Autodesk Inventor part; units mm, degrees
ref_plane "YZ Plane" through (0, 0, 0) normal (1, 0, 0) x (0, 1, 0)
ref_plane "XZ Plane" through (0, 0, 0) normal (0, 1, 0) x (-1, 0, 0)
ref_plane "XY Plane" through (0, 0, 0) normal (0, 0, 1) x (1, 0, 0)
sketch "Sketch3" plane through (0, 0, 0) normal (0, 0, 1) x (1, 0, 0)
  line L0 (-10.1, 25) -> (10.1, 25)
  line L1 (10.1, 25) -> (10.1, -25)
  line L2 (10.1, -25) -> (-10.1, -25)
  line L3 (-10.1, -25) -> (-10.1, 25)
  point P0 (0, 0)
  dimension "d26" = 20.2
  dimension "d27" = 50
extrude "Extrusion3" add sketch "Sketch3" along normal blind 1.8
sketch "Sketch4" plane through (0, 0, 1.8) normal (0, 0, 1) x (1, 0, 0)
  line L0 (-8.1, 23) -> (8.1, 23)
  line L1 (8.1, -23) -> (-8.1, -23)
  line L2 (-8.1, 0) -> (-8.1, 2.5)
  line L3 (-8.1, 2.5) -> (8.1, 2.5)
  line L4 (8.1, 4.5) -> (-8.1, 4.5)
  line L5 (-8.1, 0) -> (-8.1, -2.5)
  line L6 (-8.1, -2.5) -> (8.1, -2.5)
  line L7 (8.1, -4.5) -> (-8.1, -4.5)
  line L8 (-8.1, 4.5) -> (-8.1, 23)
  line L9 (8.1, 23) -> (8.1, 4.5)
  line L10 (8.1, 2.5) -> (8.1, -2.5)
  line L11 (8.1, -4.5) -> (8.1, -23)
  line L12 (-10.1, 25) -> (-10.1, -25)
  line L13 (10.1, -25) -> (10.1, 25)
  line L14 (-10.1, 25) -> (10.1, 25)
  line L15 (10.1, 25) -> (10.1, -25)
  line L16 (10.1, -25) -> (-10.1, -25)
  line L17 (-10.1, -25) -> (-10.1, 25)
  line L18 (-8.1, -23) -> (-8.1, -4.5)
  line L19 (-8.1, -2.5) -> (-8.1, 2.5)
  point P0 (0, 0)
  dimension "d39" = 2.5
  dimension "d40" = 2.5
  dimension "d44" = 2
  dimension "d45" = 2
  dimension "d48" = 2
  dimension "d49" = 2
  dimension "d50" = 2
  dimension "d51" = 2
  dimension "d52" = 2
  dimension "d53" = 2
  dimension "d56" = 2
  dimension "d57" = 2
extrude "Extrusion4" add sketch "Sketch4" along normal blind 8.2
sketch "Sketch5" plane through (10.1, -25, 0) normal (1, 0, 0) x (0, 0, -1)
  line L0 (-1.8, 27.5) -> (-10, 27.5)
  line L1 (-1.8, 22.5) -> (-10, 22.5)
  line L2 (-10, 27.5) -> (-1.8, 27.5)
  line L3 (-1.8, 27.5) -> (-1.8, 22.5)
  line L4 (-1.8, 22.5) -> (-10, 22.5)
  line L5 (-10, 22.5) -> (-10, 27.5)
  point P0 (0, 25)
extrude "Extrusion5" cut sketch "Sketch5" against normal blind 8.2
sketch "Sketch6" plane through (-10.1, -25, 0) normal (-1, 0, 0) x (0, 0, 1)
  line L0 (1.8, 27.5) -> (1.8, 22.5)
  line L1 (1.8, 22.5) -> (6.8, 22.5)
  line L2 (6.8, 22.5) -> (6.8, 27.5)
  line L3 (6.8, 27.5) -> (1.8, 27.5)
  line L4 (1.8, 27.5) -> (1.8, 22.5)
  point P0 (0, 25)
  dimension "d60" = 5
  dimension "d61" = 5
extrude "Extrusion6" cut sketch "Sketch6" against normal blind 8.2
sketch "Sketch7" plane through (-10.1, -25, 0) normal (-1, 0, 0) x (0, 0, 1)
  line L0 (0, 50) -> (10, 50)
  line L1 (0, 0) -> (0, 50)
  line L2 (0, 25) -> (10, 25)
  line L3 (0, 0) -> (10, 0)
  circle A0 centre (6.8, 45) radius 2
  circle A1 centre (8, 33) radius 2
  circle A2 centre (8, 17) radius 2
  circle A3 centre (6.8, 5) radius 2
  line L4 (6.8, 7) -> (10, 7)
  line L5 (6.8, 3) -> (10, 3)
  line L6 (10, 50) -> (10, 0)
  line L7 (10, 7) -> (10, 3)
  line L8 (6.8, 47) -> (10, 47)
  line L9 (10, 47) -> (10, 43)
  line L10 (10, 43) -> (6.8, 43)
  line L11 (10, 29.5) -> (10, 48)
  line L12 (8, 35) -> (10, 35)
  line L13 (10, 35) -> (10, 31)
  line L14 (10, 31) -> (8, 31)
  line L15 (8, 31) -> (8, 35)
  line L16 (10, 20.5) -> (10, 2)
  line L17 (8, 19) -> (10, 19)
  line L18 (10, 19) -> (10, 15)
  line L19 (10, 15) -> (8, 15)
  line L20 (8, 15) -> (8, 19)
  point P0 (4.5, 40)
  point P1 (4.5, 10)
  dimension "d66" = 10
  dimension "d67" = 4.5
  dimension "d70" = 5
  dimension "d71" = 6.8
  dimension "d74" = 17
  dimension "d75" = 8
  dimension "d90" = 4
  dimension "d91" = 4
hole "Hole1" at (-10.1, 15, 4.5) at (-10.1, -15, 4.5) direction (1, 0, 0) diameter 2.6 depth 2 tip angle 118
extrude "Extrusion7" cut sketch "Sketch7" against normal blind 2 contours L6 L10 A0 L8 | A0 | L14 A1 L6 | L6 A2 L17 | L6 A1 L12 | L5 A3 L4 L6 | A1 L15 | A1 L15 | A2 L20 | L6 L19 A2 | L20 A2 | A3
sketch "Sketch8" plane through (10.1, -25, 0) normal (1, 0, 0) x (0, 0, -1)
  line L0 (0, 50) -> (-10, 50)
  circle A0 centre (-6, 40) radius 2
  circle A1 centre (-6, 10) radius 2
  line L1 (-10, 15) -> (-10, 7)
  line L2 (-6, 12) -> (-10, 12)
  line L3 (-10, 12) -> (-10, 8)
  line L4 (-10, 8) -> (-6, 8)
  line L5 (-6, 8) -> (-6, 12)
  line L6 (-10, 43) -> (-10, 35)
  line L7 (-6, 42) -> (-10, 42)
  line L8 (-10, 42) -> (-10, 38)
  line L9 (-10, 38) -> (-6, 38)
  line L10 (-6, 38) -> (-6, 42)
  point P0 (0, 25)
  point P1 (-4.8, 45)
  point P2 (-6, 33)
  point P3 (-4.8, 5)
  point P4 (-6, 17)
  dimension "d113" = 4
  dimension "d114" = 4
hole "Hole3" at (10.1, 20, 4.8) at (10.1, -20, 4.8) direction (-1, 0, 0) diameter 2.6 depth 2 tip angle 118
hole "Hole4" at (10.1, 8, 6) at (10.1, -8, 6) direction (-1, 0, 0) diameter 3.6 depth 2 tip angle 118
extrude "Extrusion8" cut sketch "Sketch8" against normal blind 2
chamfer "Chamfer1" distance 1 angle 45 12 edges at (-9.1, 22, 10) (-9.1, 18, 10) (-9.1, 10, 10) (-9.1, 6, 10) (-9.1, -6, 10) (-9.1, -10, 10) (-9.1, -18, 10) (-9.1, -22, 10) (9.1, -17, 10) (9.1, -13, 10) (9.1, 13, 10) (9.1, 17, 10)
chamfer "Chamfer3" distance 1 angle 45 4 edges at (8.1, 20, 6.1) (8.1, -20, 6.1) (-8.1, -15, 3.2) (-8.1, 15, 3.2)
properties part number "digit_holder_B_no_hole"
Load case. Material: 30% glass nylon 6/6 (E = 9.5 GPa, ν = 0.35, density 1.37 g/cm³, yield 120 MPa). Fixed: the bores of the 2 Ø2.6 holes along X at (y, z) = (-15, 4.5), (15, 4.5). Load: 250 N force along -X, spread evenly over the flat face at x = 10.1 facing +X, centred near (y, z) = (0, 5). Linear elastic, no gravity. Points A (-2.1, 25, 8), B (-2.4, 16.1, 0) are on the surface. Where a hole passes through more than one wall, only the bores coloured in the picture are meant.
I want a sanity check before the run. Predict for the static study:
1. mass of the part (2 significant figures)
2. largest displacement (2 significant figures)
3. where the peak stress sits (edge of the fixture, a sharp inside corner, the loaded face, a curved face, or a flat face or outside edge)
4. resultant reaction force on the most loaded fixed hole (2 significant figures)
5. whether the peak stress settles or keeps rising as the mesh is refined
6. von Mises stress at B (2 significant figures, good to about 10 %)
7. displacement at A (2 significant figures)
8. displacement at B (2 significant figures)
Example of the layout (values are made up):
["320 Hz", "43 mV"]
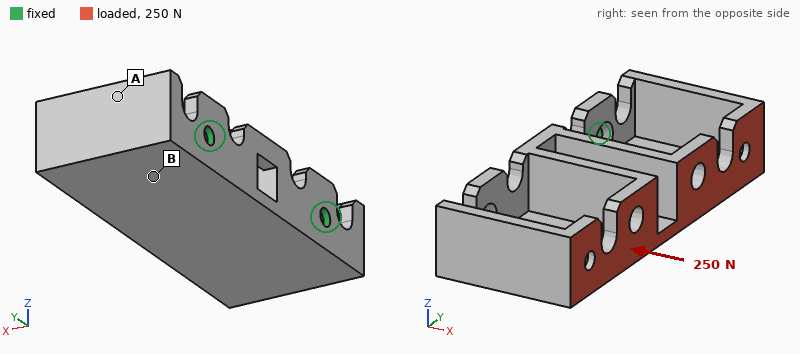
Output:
["5.5 g", "0.39 mm", "edge of the fixture", "130 N", "keeps rising", "7.1 MPa", "0.16 mm", "0.089 mm"]
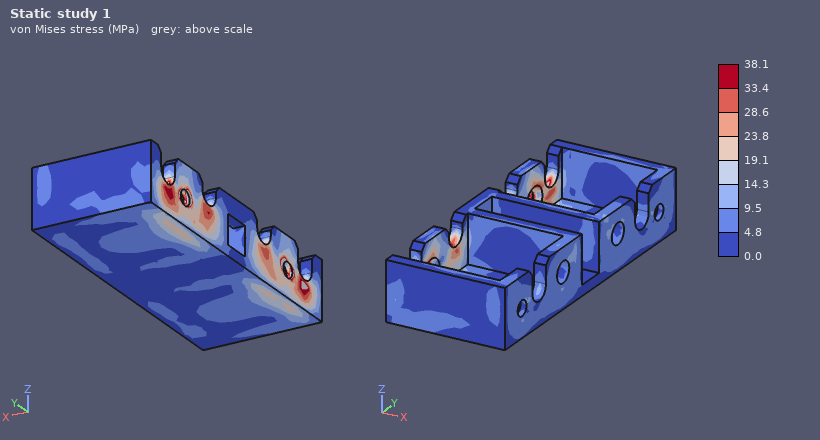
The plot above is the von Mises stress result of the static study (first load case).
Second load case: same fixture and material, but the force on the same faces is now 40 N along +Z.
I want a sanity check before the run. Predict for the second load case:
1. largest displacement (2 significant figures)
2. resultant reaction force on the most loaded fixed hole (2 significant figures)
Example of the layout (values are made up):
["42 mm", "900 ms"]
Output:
["0.59 mm", "22 N"]
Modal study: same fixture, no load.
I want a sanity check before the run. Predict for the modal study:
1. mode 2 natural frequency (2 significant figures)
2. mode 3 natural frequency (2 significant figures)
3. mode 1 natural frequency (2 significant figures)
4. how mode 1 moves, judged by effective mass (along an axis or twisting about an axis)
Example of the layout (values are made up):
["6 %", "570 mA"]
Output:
["1800 Hz", "3100 Hz", "950 Hz", "along Z"]
